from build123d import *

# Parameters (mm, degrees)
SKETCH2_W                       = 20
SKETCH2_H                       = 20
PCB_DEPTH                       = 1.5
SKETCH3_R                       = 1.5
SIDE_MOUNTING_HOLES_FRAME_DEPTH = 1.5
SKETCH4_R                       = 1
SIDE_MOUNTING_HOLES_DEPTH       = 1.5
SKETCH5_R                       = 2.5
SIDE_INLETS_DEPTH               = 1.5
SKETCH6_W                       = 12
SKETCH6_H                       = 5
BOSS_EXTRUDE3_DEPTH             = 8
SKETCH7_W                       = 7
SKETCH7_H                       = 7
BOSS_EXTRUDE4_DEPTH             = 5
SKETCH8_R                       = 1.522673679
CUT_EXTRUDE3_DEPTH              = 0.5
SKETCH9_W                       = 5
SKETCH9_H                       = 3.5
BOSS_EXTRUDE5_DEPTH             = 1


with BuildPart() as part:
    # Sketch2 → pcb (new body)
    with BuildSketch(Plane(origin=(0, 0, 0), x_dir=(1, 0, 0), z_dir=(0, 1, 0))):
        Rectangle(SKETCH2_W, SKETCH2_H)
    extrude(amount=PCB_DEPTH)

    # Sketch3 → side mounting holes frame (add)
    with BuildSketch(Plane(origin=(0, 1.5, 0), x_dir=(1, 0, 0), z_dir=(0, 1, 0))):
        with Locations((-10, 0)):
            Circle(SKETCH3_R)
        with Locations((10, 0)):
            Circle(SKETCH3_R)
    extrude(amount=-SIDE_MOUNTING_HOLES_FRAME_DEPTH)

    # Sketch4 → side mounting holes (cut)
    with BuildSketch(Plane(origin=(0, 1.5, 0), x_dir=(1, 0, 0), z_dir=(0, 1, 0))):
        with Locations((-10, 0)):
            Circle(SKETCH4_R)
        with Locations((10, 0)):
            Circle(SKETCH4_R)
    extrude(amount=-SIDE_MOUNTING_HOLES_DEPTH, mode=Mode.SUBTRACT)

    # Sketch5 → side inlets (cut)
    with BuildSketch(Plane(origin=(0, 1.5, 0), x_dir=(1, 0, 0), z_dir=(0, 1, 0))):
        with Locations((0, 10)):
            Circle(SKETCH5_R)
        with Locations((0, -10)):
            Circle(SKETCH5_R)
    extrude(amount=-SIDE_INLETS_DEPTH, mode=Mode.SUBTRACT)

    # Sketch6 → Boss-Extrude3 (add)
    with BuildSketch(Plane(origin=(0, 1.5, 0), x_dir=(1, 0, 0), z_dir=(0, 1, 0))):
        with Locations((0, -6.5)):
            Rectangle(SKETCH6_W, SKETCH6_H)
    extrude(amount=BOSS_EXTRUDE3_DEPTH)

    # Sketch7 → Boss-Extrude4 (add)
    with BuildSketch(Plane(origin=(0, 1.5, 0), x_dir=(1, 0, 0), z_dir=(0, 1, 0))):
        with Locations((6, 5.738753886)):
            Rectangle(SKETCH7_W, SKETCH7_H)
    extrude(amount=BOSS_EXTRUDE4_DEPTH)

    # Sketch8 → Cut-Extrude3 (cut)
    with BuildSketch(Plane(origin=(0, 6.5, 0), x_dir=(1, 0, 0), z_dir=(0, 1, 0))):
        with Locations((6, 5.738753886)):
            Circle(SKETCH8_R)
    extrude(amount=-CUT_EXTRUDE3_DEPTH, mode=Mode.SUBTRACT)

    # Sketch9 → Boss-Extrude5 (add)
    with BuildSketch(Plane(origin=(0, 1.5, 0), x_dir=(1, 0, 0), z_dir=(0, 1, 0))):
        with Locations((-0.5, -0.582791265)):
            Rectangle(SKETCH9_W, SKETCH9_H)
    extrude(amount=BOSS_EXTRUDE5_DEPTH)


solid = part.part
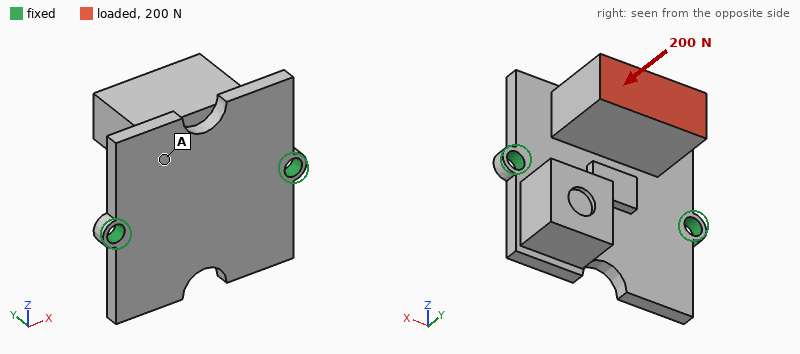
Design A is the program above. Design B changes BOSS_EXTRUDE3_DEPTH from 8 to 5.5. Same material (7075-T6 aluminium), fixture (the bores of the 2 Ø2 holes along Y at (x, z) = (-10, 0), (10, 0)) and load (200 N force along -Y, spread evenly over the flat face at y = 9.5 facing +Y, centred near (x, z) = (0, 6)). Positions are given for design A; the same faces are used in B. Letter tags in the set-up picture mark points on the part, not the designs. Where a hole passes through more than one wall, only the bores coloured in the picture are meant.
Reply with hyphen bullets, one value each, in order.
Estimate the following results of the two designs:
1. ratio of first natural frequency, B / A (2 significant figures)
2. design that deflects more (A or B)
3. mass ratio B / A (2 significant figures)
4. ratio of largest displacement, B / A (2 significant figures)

- 1.2
- A
- 0.89
- 0.87
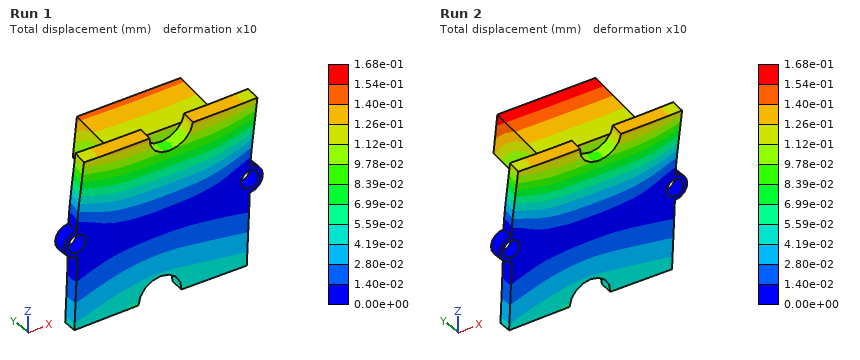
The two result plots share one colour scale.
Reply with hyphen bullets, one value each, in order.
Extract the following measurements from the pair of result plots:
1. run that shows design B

- Run 1
